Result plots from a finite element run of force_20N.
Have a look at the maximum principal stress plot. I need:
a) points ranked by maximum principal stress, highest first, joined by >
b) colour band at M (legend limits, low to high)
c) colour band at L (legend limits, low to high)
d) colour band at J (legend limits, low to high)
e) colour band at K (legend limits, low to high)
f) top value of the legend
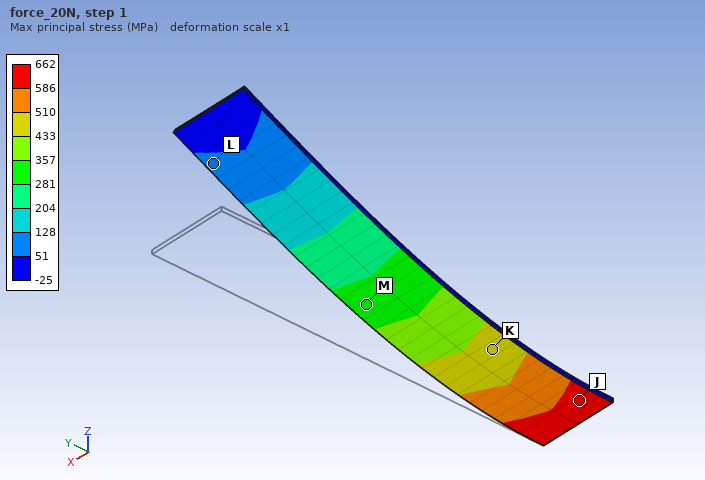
J > K > M > L
281 to 357 MPa
51 to 128 MPa
586 to 662 MPa
433 to 510 MPa
662 MPa
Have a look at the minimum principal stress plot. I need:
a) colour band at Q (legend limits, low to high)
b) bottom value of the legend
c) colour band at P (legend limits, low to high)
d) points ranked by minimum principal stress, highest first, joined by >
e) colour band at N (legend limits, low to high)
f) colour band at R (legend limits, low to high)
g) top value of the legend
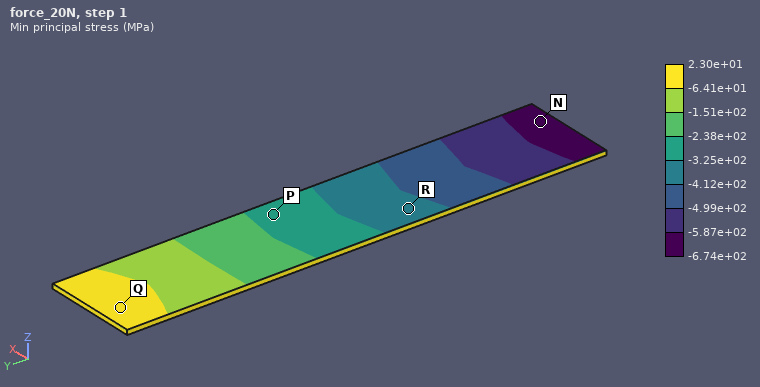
-6.41e+01 to 2.30e+01 MPa
-6.74e+02 MPa
-3.25e+02 to -2.38e+02 MPa
Q > P > R > N
-6.74e+02 to -5.87e+02 MPa
-4.12e+02 to -3.25e+02 MPa
2.30e+01 MPa
